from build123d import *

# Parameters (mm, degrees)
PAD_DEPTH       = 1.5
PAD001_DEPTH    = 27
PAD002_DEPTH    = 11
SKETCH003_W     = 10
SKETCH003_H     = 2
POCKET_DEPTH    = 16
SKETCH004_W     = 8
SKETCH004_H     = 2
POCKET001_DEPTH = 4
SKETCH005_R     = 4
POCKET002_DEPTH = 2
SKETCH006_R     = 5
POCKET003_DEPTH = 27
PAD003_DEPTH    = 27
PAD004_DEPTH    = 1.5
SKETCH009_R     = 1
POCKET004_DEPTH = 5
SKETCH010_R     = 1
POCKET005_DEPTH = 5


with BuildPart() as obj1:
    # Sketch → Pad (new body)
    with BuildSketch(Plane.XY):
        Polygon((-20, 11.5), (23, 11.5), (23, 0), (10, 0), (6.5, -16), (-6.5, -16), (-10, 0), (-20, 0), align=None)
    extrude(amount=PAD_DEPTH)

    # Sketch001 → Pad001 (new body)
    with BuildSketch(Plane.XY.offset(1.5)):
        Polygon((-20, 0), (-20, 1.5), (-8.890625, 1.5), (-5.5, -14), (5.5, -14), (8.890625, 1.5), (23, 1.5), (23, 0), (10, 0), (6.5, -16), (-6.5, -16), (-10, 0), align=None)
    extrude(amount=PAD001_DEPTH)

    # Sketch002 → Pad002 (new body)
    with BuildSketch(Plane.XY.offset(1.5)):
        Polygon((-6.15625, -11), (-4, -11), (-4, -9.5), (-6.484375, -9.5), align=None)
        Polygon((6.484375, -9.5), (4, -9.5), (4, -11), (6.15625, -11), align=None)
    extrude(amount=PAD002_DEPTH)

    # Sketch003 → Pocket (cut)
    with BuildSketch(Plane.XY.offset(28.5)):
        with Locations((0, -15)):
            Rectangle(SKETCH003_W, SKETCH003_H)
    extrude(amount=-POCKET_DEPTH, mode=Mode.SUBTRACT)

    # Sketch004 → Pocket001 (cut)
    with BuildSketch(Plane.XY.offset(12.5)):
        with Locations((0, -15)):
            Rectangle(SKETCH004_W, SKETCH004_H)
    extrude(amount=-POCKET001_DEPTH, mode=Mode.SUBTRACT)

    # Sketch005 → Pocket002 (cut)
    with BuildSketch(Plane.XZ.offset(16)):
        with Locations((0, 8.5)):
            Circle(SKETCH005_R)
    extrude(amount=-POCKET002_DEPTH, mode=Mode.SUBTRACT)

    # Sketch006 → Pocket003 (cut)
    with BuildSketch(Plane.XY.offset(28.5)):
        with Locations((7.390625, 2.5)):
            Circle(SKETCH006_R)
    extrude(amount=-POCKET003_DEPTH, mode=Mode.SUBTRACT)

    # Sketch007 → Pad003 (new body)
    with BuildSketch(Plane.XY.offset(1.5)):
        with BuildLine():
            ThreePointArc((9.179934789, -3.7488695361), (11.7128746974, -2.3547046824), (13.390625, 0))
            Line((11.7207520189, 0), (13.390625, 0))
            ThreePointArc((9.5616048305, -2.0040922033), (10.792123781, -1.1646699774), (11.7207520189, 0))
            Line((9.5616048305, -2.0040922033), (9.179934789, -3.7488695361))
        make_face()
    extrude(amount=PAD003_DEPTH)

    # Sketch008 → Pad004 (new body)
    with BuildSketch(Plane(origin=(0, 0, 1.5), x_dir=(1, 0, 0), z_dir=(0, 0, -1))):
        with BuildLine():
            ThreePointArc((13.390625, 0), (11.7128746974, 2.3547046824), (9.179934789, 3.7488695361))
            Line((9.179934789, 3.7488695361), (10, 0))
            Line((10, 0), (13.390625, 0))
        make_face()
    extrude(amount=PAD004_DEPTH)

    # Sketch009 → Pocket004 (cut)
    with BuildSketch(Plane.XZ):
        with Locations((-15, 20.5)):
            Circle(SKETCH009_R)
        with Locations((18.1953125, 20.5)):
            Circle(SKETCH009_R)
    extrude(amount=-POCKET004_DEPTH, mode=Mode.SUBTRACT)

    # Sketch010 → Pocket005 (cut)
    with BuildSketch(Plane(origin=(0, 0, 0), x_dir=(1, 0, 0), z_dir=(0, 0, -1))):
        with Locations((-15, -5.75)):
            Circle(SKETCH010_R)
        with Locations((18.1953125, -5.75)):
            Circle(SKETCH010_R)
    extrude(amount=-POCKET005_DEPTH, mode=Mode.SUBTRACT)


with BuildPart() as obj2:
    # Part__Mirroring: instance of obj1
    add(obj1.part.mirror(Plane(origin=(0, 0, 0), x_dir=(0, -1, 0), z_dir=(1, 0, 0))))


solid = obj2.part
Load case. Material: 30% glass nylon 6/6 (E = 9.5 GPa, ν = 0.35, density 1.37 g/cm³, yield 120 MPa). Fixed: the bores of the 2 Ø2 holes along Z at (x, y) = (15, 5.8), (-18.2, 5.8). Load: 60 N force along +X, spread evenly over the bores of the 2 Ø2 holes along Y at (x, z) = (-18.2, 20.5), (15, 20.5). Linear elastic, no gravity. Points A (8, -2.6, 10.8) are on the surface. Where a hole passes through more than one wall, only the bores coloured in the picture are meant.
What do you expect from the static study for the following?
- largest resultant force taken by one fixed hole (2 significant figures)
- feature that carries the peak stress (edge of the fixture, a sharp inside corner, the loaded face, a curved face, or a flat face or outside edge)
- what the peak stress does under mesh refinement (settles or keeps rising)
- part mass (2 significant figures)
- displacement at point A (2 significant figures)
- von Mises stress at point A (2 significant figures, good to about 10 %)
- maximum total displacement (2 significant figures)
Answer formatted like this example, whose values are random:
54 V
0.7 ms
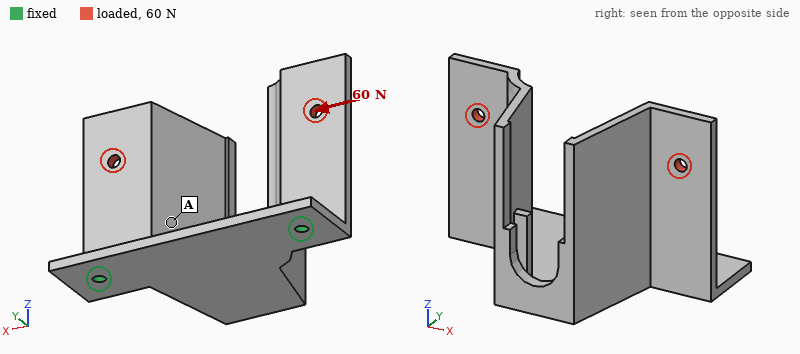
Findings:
41 N
edge of the fixture
keeps rising
4.9 g
0.15 mm
6.6 MPa
0.60 mm
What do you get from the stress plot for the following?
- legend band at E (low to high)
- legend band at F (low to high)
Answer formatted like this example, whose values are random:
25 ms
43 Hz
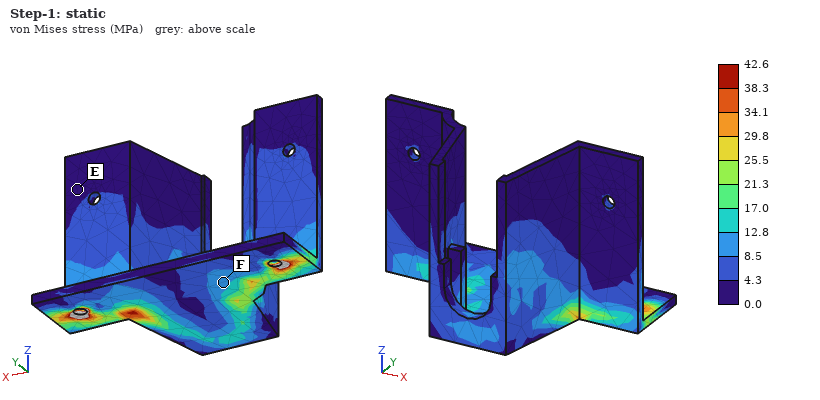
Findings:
0.0 to 4.3 MPa
8.5 to 12.8 MPa
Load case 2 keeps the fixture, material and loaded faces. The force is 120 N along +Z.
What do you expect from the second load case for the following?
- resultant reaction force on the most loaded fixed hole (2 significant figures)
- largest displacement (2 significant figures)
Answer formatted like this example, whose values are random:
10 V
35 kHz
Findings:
60 N
0.68 mm
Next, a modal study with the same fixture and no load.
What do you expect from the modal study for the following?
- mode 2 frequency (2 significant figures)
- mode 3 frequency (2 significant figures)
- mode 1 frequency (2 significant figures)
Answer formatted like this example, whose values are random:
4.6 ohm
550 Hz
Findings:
1300 Hz
1300 Hz
470 Hz
